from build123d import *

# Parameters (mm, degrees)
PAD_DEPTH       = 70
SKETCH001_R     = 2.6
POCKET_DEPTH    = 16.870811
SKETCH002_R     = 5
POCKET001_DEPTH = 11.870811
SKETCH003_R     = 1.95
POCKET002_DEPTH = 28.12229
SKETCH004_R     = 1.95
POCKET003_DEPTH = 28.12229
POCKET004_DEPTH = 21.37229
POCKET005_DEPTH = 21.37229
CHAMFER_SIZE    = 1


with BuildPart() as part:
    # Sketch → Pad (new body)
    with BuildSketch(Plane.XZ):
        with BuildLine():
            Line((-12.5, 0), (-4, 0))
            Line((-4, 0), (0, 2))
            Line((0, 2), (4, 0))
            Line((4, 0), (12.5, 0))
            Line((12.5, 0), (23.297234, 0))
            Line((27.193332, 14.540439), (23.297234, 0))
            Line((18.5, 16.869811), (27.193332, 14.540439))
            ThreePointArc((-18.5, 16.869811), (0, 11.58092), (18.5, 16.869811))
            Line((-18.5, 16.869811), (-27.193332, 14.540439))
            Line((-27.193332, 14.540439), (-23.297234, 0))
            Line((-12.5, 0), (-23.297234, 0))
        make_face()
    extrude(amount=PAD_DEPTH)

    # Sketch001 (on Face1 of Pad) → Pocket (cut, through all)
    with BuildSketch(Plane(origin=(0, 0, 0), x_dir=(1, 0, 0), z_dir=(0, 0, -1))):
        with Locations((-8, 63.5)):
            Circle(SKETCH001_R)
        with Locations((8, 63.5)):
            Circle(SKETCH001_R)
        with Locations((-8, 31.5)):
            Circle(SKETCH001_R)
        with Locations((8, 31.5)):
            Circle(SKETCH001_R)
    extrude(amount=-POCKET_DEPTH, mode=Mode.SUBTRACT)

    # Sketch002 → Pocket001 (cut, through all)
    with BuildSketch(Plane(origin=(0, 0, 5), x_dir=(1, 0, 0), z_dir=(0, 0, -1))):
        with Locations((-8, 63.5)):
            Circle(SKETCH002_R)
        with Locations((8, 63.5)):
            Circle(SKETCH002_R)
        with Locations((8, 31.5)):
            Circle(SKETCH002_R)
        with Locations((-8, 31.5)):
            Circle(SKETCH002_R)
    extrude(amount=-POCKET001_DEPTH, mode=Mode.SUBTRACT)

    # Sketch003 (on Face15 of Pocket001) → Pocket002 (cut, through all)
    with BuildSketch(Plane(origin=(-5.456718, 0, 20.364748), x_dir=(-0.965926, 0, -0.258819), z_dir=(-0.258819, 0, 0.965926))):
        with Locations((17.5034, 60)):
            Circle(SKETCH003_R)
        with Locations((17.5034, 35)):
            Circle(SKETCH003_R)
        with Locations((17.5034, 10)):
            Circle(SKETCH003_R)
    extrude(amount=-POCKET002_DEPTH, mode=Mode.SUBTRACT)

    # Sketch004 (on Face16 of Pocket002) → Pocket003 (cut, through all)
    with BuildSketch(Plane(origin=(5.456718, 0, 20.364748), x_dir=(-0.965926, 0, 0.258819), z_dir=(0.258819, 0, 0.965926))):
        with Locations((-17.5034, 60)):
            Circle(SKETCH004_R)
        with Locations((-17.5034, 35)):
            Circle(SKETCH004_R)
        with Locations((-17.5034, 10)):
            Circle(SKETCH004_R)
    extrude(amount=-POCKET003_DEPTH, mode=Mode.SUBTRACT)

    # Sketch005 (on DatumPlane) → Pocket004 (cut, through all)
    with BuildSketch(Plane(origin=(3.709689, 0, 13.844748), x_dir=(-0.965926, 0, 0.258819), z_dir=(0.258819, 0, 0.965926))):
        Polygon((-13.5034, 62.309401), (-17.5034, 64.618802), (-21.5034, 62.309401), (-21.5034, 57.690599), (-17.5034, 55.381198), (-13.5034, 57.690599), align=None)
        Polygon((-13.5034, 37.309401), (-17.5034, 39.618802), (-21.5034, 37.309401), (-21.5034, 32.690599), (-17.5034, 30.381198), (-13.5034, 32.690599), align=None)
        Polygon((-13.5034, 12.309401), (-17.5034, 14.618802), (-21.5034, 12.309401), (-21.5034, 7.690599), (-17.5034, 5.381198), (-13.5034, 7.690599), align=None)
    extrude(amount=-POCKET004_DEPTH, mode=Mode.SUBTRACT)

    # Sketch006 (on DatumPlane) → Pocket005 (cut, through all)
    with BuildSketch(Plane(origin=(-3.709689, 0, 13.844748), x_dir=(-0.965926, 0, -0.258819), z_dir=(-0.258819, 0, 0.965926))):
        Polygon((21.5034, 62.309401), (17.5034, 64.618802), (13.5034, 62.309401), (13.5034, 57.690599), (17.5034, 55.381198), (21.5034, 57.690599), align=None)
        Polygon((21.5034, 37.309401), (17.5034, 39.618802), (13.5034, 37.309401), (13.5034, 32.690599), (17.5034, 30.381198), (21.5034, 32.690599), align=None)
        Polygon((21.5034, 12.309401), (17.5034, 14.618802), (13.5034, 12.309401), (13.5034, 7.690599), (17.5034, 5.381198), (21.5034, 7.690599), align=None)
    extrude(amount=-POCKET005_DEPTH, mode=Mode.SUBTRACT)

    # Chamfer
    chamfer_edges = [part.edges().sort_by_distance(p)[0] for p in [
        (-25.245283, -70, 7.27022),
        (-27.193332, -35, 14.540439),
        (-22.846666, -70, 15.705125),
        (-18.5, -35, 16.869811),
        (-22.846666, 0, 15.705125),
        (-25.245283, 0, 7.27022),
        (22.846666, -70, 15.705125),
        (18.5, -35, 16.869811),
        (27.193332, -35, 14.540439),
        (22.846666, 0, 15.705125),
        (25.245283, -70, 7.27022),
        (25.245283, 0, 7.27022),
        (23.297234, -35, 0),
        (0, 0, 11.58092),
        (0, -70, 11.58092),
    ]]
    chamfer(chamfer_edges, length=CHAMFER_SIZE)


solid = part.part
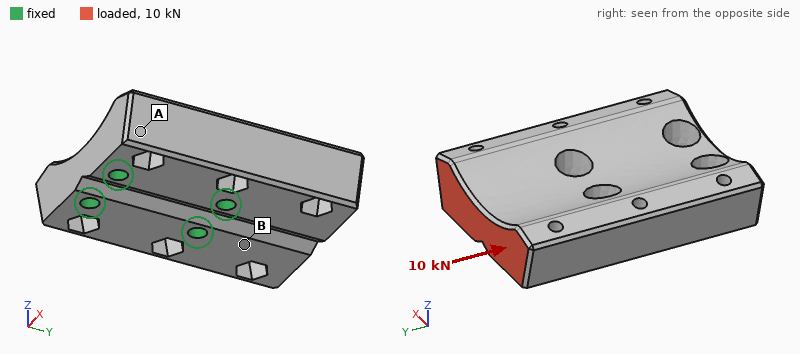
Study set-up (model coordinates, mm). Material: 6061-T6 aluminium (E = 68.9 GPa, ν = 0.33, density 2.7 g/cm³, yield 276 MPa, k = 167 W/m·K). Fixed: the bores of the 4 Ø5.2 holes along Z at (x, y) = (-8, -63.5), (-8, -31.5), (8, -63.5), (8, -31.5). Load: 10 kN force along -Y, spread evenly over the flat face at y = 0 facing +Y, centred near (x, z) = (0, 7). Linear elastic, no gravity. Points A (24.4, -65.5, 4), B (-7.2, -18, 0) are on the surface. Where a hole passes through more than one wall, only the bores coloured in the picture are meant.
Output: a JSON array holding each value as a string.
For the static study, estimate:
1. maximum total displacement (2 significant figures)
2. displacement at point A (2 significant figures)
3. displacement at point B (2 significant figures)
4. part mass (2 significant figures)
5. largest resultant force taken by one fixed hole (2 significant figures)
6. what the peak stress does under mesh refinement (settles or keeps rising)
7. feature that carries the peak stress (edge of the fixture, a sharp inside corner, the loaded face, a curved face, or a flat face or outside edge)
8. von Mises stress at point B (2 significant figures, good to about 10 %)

["20 µm", "4.2 µm", "8.0 µm", "110 g", "3.7 kN", "keeps rising", "edge of the fixture", "29 MPa"]
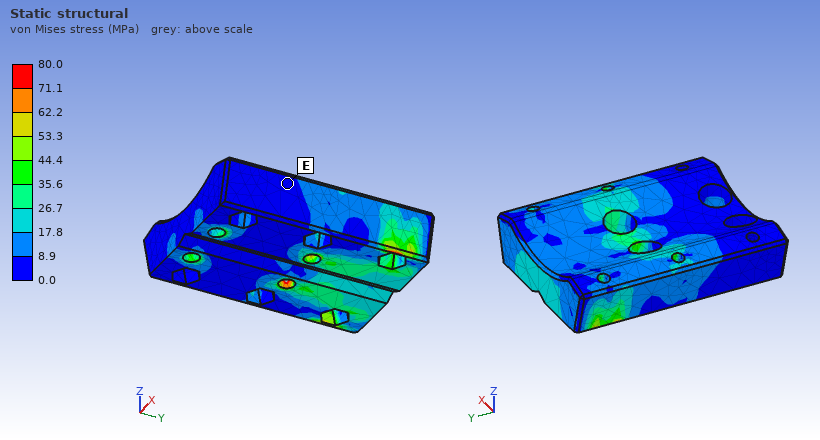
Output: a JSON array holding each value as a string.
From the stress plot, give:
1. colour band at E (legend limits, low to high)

["0.0 to 8.9 MPa"]
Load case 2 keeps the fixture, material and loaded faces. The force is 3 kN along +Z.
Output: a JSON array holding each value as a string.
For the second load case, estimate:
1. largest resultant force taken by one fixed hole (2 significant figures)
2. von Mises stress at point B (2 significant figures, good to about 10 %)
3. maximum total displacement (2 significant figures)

["3.2 kN", "35 MPa", "0.10 mm"]
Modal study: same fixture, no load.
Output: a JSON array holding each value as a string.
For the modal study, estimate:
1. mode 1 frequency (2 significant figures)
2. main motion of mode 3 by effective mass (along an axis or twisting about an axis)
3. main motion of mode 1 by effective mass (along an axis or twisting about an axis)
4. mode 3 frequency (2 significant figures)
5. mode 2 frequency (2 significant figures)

["6700 Hz", "along X", "along Z", "12 kHz", "8100 Hz"]
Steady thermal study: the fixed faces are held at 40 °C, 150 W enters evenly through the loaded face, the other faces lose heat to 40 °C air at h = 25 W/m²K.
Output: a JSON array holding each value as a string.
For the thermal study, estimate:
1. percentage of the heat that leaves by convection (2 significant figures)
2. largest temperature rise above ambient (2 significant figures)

["3.8 %", "62 K"]
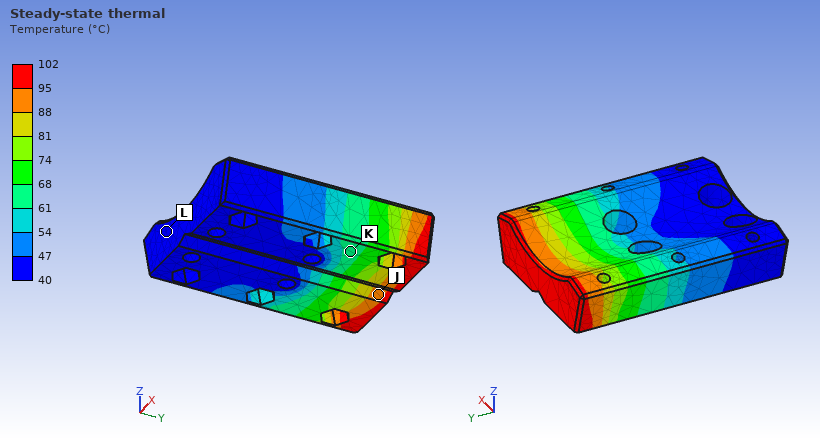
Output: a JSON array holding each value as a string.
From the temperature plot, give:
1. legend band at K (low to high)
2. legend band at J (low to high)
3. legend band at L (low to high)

["61 to 68 °C", "88 to 95 °C", "40 to 47 °C"]
